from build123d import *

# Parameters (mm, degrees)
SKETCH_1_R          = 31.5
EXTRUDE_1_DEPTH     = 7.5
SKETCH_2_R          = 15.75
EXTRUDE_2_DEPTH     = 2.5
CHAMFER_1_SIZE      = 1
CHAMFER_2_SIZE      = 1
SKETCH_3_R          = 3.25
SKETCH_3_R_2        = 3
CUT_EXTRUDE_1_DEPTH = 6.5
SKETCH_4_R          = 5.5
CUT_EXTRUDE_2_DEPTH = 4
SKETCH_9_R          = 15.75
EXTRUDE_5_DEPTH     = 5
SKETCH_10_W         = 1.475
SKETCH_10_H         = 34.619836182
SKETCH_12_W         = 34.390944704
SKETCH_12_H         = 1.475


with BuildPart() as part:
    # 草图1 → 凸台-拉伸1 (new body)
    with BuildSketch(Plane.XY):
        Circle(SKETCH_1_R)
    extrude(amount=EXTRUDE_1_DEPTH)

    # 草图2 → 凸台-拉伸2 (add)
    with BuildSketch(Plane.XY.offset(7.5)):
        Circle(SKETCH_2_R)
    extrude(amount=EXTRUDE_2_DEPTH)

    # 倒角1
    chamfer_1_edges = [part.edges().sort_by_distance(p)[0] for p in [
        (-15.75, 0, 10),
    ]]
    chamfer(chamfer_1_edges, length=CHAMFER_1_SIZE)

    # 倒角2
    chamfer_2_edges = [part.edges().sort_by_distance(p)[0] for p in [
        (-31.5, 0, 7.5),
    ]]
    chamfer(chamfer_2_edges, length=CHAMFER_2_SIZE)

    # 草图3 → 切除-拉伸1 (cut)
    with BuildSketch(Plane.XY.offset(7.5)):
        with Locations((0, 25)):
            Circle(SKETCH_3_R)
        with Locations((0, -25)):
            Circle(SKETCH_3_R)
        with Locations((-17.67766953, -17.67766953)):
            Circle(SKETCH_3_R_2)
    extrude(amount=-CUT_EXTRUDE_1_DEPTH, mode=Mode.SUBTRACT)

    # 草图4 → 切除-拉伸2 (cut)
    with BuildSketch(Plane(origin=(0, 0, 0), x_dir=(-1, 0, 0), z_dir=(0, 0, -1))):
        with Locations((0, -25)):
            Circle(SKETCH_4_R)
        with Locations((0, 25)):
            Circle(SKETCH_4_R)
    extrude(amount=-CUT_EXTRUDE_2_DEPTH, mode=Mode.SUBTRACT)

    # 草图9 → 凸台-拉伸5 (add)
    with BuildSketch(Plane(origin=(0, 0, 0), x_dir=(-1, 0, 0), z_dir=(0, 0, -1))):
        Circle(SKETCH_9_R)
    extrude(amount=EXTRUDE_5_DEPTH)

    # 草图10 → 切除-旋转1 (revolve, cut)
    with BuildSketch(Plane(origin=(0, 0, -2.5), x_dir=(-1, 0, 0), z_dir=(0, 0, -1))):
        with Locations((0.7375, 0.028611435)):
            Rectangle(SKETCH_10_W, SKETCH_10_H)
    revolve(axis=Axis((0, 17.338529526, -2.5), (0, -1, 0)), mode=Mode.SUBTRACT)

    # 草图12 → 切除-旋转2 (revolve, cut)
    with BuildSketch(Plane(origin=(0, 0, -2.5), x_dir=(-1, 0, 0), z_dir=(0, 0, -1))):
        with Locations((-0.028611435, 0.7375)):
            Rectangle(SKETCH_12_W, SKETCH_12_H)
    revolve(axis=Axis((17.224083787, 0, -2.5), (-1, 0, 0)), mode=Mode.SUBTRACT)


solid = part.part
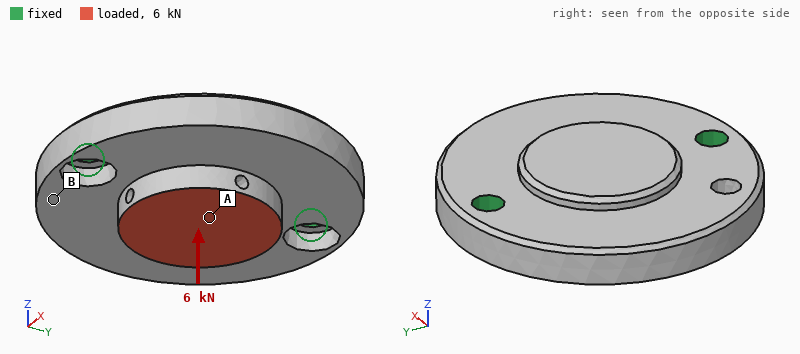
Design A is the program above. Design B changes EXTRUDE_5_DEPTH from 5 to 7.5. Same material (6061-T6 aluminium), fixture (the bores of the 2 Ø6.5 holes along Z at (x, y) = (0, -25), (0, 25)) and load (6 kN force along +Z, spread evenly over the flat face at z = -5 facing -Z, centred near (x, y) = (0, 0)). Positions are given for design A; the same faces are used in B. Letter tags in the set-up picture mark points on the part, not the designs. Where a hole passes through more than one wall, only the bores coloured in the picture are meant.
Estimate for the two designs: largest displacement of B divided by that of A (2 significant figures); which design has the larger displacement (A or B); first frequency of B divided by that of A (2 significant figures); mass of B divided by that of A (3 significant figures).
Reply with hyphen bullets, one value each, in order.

- 0.86
- A
- 0.97
- 1.07
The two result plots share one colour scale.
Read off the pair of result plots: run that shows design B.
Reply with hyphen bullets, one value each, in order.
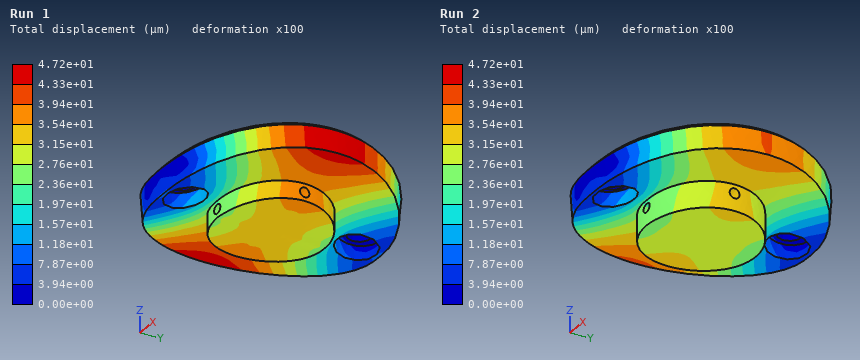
- Run 2
